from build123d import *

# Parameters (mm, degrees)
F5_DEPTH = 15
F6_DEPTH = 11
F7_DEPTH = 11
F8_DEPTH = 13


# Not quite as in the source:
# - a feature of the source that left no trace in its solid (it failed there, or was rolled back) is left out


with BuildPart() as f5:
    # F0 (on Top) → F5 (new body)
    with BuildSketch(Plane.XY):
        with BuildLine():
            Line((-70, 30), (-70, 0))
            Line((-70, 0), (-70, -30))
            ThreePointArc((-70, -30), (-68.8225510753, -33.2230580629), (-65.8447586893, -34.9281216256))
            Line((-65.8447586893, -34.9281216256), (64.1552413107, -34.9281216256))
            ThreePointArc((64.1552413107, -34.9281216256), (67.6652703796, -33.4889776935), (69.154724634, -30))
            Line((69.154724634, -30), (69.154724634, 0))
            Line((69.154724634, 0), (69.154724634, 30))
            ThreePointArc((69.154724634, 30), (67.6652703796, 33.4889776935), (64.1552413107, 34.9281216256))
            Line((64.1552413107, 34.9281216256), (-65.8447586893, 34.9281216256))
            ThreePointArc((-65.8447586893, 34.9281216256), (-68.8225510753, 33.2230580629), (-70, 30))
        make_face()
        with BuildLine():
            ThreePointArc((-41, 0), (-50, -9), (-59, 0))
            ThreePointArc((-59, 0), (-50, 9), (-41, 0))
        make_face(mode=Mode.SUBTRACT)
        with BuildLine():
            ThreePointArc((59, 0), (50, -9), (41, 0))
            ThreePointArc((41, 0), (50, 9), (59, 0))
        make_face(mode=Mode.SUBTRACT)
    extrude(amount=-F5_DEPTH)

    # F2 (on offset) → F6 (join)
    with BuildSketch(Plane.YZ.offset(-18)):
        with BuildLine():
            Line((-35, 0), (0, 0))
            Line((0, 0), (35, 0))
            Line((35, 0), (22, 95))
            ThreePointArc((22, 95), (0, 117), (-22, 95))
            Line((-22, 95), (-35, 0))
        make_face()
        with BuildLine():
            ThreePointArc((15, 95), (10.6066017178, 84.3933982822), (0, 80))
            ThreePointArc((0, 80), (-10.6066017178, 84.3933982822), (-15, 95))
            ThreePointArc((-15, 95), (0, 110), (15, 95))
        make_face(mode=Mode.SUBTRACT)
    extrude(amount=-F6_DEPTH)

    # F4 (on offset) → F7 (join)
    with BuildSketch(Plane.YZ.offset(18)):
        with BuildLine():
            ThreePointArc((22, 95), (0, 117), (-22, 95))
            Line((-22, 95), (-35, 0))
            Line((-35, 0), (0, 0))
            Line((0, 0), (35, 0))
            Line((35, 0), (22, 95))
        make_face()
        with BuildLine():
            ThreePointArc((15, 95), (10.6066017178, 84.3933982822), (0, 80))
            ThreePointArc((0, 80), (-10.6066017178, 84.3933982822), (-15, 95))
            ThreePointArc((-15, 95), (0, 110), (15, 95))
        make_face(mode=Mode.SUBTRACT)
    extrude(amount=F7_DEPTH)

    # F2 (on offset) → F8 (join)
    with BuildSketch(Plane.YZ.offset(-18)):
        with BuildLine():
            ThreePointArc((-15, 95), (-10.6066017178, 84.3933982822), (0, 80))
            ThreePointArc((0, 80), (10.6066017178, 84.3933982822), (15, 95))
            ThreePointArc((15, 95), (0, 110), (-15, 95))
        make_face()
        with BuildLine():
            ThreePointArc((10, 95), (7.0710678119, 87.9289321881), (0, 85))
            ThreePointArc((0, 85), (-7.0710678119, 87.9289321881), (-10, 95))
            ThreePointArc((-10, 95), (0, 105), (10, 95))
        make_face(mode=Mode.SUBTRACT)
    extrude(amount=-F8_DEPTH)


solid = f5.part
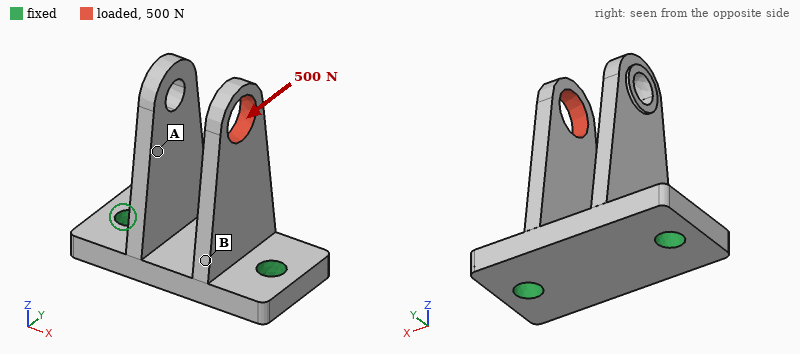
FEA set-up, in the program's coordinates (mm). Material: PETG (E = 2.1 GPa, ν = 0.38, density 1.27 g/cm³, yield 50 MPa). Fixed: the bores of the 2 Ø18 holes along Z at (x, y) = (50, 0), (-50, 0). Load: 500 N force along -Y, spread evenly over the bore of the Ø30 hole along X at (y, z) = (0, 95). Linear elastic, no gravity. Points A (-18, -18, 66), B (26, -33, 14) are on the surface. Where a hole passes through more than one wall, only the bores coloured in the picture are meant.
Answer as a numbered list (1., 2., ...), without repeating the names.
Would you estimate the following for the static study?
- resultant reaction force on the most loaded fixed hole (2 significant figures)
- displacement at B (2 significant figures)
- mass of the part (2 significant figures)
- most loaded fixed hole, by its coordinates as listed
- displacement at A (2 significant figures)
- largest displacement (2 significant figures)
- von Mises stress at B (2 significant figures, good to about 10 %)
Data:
1. 390 N
2. 0.47 mm
3. 330 g
4. (50, 0)
5. 0.38 mm
6. 2.1 mm
7. 5.2 MPa
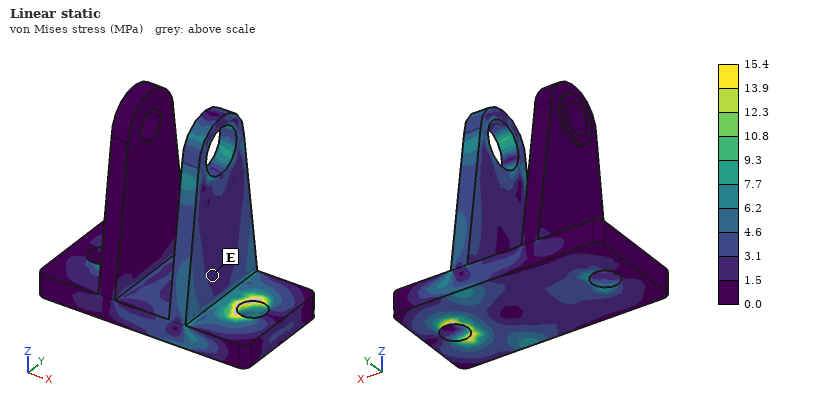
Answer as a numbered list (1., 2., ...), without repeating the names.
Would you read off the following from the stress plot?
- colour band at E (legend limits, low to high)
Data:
1. 1.5 to 3.1 MPa
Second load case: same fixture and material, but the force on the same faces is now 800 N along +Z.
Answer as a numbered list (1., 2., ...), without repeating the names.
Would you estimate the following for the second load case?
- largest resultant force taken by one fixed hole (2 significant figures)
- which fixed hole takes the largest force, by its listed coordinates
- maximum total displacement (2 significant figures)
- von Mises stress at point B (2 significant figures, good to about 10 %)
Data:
1. 660 N
2. (50, 0)
3. 0.29 mm
4. 0.49 MPa
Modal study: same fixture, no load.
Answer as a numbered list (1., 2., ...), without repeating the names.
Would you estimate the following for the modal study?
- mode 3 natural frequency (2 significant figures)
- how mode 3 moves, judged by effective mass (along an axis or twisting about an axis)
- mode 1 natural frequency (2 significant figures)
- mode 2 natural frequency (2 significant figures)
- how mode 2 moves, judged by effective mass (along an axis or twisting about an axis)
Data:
1. 440 Hz
2. along Y
3. 210 Hz
4. 240 Hz
5. along X
